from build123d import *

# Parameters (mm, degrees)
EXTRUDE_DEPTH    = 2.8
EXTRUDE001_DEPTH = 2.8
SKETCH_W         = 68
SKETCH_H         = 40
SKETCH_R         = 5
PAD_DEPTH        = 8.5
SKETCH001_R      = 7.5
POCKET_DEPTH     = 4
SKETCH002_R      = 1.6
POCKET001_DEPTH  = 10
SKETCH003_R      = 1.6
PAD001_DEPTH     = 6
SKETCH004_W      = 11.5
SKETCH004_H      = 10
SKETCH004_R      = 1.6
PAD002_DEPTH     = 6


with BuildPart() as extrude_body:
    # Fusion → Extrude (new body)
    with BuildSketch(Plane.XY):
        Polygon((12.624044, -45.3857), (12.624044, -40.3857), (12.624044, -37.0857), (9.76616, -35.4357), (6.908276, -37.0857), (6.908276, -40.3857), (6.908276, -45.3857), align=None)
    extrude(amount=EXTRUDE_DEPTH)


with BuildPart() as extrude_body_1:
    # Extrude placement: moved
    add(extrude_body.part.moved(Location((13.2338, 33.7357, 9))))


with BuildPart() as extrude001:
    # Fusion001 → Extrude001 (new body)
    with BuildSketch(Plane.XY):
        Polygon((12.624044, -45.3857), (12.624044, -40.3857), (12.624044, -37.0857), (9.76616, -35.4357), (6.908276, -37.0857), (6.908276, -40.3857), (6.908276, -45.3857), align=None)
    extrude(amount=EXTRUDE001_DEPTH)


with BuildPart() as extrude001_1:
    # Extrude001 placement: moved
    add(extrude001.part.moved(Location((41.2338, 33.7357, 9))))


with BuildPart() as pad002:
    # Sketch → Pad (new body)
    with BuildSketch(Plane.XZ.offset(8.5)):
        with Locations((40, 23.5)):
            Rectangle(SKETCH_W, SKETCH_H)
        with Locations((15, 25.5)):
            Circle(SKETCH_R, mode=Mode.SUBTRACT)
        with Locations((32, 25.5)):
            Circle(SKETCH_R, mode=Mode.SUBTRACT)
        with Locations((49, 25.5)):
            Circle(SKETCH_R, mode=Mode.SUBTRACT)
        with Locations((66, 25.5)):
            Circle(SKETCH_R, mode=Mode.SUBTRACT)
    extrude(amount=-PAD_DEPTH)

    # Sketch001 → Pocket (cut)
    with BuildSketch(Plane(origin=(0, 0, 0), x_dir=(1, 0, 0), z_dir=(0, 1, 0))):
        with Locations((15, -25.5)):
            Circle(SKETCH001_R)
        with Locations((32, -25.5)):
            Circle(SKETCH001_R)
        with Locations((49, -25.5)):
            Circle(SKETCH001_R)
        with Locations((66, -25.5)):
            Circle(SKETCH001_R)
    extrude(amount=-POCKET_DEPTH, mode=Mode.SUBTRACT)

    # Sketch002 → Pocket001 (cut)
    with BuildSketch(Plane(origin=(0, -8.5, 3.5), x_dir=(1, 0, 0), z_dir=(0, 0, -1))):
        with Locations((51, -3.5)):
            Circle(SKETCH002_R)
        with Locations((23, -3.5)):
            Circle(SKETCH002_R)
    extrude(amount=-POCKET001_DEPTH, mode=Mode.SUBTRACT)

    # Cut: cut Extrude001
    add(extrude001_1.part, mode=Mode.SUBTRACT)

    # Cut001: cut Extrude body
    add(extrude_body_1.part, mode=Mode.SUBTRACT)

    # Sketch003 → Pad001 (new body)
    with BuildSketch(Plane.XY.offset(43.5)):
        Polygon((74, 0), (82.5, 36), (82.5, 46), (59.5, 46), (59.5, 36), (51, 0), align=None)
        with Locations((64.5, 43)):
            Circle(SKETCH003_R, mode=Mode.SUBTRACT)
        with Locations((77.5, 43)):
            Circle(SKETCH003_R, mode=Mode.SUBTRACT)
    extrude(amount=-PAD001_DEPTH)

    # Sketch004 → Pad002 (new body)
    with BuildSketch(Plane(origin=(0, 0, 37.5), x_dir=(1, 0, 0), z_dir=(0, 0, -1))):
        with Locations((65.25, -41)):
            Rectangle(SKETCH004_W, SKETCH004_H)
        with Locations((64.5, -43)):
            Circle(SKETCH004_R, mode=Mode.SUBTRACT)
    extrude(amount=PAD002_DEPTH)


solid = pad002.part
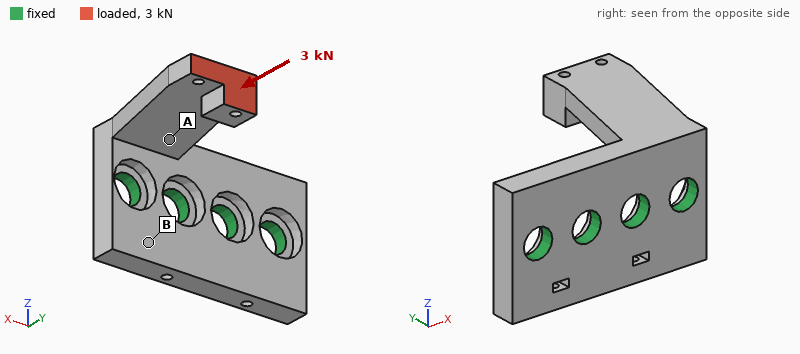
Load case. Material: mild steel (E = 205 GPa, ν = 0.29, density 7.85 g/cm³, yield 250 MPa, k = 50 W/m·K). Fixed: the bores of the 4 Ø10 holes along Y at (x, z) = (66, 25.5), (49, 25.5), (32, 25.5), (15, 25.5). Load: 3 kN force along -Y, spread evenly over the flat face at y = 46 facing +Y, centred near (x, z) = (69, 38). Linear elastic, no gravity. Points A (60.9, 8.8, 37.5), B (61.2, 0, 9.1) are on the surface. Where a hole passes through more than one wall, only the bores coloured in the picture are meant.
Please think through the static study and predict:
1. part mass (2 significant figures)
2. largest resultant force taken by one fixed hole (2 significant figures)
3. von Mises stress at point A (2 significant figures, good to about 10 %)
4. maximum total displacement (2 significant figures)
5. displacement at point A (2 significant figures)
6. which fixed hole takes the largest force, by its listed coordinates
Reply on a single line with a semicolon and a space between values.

200 g; 3.1 kN; 55 MPa; 68 µm; 22 µm; (66, 25.5)
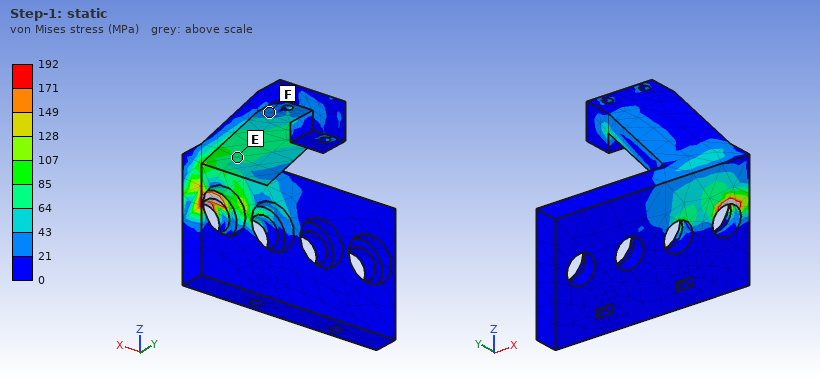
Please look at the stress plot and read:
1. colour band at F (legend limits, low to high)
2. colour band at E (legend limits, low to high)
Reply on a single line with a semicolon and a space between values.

21 to 43 MPa; 64 to 85 MPa
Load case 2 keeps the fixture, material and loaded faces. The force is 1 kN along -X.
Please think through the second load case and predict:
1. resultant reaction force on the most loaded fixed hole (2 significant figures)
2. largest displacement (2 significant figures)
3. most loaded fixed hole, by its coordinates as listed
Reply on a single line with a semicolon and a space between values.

2.3 kN; 0.12 mm; (66, 25.5)
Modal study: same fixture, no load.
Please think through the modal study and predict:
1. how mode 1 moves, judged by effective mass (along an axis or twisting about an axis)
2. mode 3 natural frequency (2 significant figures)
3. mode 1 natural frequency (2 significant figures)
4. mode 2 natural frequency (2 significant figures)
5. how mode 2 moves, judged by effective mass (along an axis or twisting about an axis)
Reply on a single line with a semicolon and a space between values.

along Z; 7300 Hz; 1500 Hz; 3500 Hz; along X
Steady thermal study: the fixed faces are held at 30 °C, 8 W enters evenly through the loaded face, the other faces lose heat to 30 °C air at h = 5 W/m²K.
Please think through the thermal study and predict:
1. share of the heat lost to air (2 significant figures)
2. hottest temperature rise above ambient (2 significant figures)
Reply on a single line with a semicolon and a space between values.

7.8 %; 63 K
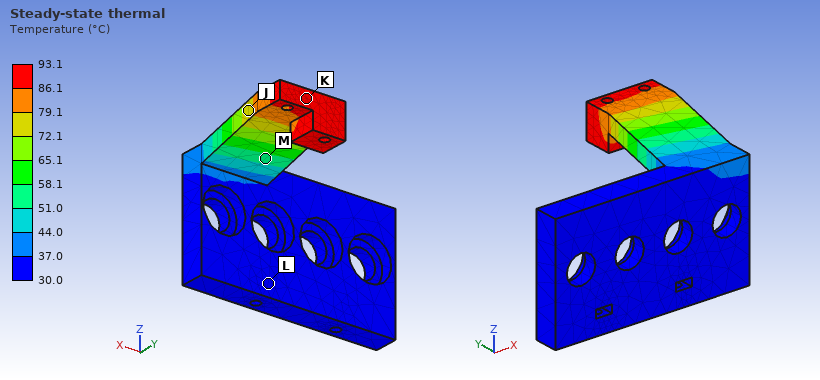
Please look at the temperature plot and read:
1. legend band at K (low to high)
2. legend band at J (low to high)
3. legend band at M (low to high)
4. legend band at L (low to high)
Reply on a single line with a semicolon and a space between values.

86.1 to 93.1 °C; 72.1 to 79.1 °C; 51.0 to 58.1 °C; 30.0 to 37.0 °C
